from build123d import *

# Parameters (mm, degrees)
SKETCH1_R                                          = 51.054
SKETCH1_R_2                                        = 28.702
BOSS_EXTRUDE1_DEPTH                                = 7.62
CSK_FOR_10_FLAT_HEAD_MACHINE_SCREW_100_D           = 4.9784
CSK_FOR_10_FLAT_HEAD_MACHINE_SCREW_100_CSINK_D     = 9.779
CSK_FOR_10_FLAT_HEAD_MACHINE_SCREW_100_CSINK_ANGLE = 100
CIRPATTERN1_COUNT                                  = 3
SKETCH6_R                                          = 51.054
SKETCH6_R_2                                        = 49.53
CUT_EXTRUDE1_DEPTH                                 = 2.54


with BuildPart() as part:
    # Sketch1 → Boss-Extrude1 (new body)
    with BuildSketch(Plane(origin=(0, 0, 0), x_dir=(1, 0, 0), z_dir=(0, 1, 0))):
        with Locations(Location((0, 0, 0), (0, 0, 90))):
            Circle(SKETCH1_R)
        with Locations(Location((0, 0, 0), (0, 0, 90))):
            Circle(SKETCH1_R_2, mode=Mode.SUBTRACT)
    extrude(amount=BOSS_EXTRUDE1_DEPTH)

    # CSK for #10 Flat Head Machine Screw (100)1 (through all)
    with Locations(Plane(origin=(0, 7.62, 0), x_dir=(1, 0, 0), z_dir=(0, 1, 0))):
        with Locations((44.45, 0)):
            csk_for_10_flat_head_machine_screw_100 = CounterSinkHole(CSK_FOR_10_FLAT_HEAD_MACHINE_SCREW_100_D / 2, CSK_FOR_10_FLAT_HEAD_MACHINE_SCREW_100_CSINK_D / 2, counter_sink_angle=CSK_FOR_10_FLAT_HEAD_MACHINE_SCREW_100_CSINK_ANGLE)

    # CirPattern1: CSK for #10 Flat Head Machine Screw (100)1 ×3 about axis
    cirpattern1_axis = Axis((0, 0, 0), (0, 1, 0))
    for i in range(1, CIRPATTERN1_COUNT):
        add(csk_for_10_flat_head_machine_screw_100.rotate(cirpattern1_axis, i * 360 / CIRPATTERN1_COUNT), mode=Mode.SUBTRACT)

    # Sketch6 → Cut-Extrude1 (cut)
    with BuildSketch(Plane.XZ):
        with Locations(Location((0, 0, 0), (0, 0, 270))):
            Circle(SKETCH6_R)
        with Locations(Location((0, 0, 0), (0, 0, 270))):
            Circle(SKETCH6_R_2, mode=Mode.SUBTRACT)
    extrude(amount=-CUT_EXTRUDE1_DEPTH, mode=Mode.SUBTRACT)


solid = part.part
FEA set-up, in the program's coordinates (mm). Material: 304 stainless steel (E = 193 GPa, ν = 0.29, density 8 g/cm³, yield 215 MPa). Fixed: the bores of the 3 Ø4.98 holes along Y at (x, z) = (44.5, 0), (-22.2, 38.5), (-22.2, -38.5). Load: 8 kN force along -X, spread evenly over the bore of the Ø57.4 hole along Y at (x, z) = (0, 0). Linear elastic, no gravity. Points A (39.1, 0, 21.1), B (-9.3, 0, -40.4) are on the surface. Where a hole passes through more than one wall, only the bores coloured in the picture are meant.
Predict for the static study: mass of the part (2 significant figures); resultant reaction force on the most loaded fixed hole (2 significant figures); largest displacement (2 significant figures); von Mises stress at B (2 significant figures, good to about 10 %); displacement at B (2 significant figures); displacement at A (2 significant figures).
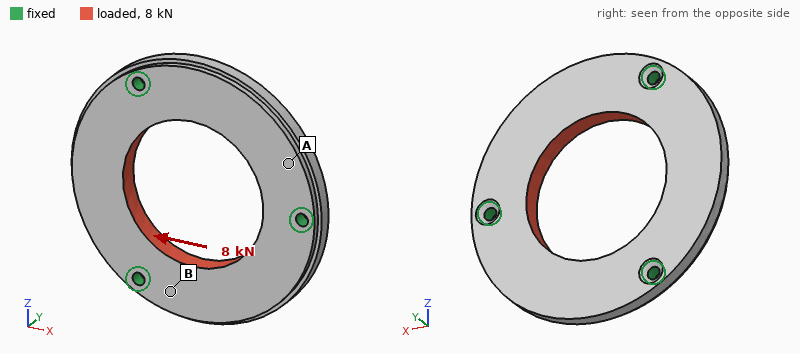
330 g
3.2 kN
5.5 µm
16 MPa
1.4 µm
2.1 µm
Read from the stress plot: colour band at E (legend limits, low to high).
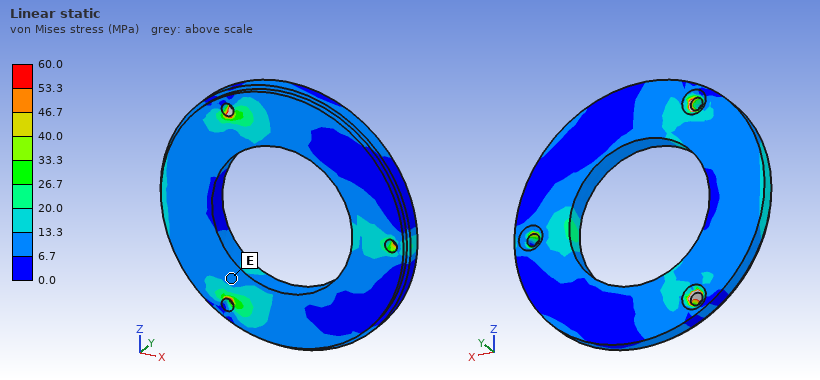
6.7 to 13.3 MPa
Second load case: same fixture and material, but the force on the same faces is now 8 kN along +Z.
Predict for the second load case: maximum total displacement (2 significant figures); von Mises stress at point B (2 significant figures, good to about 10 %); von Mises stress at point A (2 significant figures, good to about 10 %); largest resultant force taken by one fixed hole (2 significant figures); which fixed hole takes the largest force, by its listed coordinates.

4.8 µm
8.3 MPa
12 MPa
3.5 kN
(44.5, 0)
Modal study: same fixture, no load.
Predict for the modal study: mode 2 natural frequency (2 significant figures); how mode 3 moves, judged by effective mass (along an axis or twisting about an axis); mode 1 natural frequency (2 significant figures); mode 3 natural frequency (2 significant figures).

3600 Hz
along Y
3600 Hz
4300 Hz
